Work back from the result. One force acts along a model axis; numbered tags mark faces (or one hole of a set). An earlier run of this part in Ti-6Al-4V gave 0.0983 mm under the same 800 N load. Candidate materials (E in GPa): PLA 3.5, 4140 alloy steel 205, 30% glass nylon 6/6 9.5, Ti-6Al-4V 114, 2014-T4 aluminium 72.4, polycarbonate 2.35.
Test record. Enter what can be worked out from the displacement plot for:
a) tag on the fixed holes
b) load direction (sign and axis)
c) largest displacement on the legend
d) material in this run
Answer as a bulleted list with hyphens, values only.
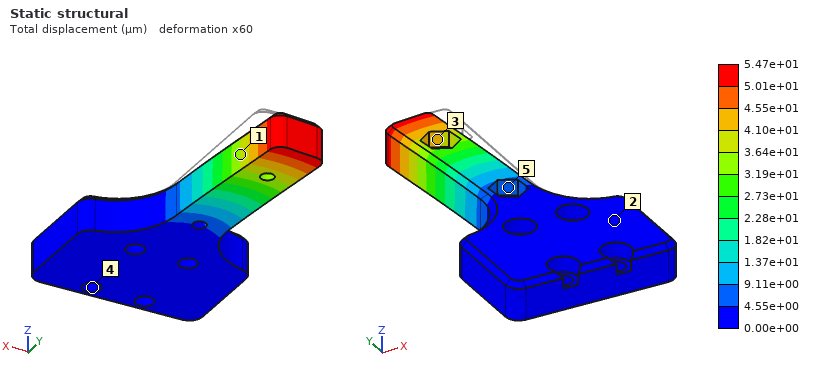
- 4
- -X
- 5.47e+01 µm
- 4140 alloy steel
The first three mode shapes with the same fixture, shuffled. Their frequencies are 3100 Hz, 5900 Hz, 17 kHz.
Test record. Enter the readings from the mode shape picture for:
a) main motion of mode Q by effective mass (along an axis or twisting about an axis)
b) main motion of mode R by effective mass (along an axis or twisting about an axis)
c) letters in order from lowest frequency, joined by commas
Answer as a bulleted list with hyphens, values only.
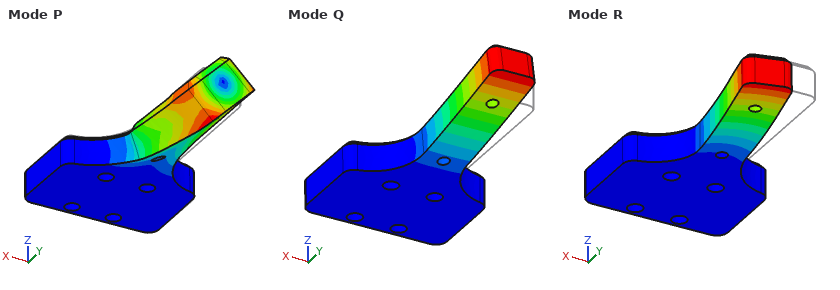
- along Z
- along X
- Q, R, P
